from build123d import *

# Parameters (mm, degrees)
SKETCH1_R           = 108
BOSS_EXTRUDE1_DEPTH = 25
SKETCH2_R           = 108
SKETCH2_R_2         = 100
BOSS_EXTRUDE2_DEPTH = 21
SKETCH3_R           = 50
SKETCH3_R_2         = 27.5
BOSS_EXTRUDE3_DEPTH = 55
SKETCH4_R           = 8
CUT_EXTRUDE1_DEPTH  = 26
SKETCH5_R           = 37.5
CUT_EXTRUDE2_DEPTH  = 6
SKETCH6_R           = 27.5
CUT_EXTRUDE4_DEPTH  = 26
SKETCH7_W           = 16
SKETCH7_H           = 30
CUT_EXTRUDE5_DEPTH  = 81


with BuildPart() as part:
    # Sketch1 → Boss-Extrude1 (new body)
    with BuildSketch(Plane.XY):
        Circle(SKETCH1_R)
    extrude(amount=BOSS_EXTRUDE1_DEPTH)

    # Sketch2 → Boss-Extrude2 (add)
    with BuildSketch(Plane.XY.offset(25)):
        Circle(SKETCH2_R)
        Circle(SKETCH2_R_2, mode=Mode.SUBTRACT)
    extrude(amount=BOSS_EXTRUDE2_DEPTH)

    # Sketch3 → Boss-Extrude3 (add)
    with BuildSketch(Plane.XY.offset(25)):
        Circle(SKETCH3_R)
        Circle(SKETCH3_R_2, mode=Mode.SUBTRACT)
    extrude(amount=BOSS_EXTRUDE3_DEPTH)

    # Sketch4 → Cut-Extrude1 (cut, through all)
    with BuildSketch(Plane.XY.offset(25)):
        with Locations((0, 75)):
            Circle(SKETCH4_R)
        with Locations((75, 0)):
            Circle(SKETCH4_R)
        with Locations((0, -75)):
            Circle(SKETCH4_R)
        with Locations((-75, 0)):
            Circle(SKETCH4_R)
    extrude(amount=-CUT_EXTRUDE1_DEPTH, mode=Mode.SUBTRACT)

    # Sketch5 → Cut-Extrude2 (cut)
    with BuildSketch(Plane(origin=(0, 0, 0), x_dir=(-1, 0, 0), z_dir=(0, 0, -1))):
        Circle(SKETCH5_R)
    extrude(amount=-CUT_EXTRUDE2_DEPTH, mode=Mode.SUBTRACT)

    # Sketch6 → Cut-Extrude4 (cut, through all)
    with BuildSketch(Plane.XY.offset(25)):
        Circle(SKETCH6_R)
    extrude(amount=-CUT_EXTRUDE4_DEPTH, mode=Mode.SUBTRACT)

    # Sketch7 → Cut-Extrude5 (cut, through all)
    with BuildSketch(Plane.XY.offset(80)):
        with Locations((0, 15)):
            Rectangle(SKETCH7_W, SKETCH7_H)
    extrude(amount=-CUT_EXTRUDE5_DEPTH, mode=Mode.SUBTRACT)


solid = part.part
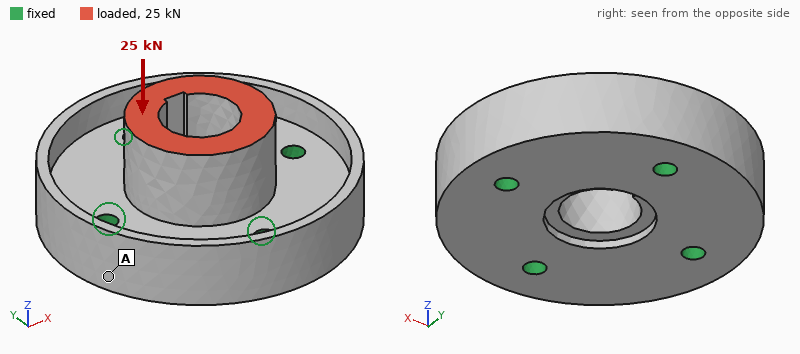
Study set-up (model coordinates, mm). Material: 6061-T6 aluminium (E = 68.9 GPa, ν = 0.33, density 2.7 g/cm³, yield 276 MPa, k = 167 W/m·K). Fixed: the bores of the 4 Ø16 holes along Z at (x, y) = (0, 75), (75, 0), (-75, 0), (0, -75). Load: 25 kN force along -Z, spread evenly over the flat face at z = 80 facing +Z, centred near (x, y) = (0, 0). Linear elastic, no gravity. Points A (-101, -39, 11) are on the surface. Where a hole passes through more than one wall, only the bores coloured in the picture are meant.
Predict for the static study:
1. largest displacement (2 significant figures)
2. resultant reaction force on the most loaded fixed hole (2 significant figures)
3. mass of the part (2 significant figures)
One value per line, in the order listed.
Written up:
14 µm
6.7 kN
3.3 kg
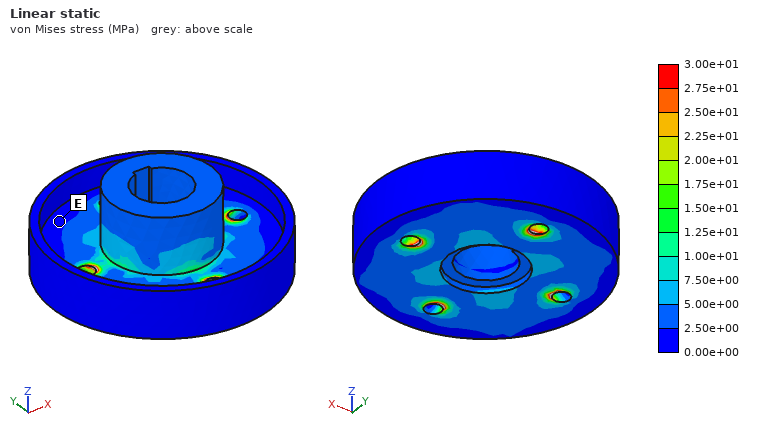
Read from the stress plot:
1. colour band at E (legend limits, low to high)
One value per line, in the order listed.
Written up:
0.00e+00 to 2.50e+00 MPa
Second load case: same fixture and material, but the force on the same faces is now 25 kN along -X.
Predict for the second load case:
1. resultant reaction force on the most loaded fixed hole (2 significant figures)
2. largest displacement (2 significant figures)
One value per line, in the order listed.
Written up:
14 kN
56 µm
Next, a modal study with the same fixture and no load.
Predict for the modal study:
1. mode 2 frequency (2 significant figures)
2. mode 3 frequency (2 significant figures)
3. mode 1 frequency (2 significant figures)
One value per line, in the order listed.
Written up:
5200 Hz
5200 Hz
4800 Hz
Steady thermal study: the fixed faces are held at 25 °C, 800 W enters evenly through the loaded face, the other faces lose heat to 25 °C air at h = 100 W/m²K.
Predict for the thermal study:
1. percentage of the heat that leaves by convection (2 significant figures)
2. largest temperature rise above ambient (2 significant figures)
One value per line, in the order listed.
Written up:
24 %
67 K
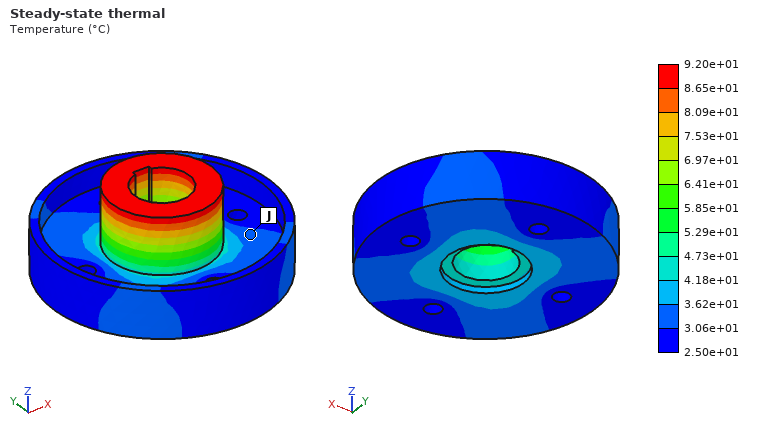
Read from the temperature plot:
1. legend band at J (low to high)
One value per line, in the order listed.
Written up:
3.06e+01 to 3.62e+01 °C
